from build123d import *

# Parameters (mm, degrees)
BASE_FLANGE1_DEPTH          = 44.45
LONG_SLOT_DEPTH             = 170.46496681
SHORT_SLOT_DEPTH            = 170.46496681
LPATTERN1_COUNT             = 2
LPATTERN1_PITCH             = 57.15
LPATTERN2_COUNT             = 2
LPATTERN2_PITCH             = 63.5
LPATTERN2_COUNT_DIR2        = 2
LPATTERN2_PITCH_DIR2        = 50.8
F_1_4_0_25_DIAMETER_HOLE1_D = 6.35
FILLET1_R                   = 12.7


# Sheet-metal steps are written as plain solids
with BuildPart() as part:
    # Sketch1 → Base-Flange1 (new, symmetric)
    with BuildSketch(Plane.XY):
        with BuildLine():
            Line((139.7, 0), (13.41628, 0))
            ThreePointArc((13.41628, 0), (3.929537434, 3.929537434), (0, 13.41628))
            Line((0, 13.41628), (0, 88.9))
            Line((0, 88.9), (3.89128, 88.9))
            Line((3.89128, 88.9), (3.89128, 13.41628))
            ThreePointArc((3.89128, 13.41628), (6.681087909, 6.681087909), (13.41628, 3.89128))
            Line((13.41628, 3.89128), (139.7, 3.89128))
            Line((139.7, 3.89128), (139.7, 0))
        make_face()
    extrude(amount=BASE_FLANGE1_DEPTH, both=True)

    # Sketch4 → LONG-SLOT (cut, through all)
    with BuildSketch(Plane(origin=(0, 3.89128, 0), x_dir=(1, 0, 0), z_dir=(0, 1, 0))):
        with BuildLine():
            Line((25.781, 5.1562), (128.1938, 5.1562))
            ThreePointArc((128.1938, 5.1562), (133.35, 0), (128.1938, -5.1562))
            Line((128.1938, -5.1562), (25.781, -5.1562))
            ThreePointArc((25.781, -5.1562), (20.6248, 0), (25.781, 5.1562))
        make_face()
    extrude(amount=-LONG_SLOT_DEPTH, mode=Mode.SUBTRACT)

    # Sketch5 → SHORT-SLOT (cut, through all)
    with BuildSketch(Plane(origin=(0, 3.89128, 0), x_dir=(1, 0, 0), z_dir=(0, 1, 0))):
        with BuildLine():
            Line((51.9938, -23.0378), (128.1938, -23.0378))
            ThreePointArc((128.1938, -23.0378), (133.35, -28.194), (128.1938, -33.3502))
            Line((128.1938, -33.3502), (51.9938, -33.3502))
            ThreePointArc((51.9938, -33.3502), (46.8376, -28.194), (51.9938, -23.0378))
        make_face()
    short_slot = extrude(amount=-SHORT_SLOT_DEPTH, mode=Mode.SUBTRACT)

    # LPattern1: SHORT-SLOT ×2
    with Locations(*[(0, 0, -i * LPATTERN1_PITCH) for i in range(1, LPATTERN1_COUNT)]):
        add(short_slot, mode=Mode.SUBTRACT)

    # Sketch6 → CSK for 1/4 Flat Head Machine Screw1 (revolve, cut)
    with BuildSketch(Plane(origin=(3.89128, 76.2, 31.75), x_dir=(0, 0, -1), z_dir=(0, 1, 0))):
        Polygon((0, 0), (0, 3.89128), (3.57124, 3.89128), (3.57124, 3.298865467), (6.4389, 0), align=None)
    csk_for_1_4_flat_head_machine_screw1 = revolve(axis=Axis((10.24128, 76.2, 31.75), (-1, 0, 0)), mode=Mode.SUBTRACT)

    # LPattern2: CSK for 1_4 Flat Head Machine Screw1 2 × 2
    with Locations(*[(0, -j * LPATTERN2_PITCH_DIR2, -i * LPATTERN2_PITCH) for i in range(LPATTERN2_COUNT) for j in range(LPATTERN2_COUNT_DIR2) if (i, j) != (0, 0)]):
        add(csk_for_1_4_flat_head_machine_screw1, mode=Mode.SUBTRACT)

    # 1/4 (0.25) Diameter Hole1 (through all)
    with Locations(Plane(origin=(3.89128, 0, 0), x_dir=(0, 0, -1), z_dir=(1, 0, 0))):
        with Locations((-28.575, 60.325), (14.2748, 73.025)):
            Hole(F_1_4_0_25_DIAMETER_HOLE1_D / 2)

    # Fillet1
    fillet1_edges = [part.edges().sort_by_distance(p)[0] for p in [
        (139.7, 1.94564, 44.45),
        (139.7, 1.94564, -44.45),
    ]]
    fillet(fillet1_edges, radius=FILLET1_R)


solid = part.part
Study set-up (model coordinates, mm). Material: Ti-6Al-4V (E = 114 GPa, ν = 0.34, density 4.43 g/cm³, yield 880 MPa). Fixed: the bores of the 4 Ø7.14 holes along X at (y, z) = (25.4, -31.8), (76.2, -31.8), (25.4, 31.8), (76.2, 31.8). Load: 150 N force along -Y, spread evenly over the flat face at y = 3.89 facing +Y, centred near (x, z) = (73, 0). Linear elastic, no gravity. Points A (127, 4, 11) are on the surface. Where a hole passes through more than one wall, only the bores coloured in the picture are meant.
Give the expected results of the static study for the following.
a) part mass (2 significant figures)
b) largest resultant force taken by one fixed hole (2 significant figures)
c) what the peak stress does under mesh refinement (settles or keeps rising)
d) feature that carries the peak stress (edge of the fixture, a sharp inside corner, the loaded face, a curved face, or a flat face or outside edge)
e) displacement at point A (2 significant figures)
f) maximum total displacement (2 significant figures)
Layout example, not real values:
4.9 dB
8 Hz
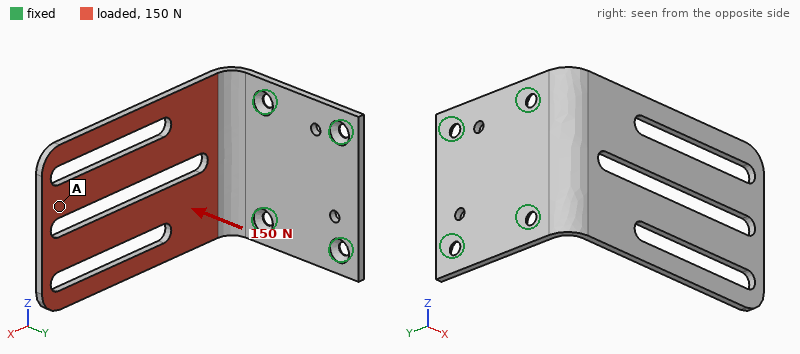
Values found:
280 g
520 N
keeps rising
edge of the fixture
1.6 mm
1.8 mm
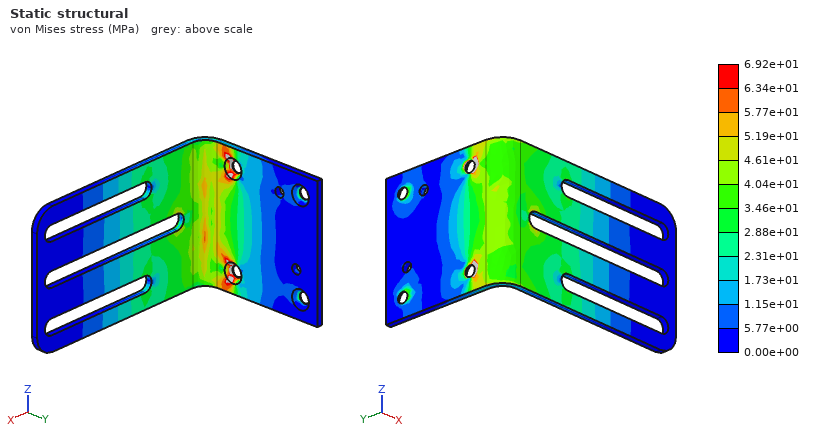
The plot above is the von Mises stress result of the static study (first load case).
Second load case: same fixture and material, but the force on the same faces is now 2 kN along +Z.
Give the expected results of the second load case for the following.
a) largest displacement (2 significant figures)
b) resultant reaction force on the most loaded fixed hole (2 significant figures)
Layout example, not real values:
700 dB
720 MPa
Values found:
2.0 mm
4.2 kN
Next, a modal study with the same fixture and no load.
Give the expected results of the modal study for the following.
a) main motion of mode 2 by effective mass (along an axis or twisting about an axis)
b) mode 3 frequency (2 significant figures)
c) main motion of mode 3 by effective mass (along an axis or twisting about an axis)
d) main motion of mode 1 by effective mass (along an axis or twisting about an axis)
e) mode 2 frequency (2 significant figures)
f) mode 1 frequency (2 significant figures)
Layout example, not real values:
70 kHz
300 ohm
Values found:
along Z
640 Hz
along Z
along Y
440 Hz
150 Hz
